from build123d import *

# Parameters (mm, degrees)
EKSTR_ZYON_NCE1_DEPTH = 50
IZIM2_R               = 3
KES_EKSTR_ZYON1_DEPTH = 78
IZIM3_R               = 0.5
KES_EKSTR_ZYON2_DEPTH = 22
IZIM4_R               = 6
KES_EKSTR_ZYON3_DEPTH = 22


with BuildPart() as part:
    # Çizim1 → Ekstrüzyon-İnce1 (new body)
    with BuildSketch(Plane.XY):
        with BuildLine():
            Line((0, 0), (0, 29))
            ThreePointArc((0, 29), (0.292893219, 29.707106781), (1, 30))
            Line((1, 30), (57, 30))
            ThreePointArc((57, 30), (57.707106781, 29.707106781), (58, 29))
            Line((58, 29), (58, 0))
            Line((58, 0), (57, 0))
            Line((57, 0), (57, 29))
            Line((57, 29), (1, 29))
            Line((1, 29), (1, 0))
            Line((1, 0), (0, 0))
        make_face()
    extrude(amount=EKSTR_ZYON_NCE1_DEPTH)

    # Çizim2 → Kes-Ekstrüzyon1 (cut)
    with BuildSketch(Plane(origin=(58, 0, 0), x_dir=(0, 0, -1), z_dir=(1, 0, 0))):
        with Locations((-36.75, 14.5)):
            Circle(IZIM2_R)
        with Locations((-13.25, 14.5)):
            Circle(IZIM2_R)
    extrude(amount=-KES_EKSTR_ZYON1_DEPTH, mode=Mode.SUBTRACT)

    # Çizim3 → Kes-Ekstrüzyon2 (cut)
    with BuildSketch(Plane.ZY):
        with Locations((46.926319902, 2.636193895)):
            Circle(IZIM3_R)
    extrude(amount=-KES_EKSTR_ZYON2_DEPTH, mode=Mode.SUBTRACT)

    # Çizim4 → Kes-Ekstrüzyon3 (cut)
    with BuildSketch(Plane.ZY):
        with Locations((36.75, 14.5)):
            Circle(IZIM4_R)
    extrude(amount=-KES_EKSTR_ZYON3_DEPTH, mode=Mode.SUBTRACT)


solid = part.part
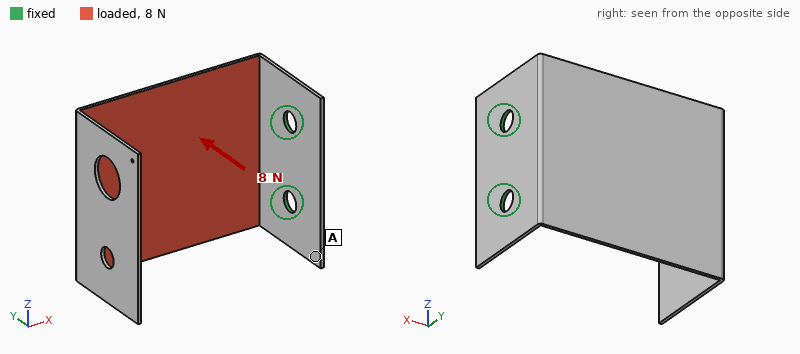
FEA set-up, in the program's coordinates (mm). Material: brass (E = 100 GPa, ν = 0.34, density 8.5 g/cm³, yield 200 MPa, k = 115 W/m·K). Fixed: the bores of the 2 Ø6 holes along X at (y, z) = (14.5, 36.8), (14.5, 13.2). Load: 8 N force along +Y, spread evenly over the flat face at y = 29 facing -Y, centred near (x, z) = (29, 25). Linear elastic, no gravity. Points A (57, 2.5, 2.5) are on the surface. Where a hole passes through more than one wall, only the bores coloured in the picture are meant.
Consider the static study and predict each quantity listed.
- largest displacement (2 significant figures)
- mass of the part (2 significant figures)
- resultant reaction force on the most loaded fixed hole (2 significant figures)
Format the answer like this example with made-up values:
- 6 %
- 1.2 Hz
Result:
- 0.90 mm
- 47 g
- 4.2 N
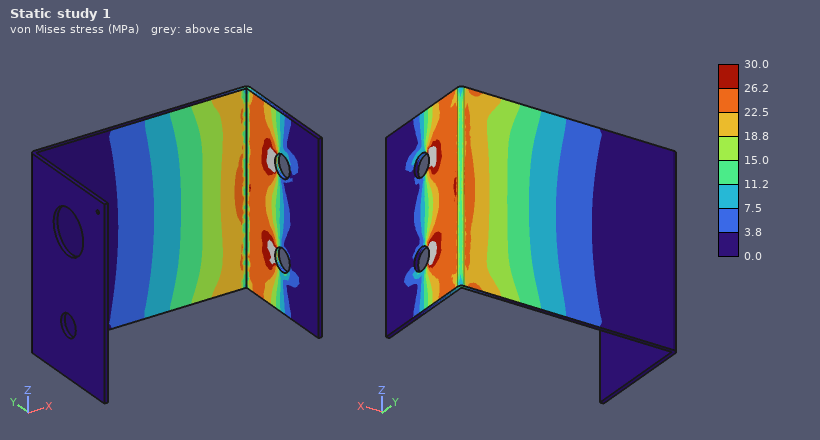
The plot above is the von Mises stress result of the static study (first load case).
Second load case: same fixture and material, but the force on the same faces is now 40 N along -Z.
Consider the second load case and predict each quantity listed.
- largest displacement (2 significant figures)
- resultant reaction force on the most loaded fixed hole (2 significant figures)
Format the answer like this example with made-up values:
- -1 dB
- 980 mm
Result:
- 0.58 mm
- 47 N
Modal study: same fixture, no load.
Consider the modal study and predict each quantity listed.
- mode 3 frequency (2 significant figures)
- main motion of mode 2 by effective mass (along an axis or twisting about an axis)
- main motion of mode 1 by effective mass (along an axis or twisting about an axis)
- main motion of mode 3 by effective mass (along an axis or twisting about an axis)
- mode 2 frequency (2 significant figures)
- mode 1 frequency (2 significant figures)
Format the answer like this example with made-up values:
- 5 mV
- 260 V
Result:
- 320 Hz
- along Z
- along Y
- along X
- 180 Hz
- 75 Hz
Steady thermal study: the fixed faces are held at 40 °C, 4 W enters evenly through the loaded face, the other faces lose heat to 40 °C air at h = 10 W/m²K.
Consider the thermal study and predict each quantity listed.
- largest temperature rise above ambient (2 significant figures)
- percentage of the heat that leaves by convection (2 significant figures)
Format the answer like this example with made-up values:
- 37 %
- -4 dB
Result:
- 20 K
- 27 %
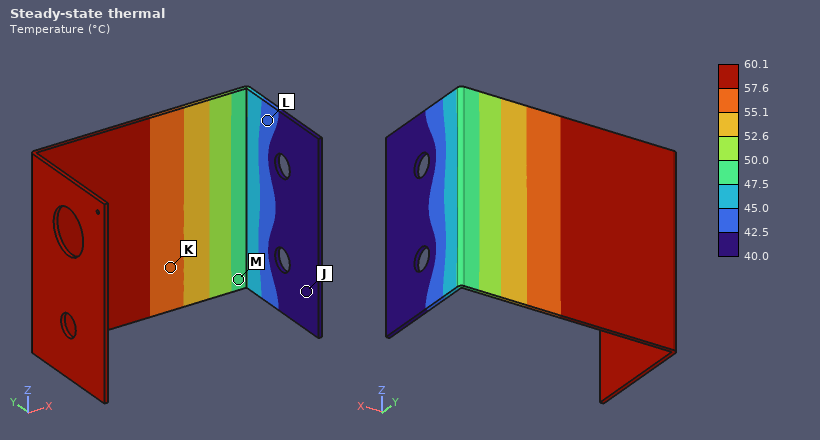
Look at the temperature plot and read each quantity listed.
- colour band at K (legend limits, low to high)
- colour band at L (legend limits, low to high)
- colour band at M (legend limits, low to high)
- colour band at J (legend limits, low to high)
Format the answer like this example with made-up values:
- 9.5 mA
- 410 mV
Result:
- 55.1 to 57.6 °C
- 42.5 to 45.0 °C
- 47.5 to 50.0 °C
- 40.0 to 42.5 °C
